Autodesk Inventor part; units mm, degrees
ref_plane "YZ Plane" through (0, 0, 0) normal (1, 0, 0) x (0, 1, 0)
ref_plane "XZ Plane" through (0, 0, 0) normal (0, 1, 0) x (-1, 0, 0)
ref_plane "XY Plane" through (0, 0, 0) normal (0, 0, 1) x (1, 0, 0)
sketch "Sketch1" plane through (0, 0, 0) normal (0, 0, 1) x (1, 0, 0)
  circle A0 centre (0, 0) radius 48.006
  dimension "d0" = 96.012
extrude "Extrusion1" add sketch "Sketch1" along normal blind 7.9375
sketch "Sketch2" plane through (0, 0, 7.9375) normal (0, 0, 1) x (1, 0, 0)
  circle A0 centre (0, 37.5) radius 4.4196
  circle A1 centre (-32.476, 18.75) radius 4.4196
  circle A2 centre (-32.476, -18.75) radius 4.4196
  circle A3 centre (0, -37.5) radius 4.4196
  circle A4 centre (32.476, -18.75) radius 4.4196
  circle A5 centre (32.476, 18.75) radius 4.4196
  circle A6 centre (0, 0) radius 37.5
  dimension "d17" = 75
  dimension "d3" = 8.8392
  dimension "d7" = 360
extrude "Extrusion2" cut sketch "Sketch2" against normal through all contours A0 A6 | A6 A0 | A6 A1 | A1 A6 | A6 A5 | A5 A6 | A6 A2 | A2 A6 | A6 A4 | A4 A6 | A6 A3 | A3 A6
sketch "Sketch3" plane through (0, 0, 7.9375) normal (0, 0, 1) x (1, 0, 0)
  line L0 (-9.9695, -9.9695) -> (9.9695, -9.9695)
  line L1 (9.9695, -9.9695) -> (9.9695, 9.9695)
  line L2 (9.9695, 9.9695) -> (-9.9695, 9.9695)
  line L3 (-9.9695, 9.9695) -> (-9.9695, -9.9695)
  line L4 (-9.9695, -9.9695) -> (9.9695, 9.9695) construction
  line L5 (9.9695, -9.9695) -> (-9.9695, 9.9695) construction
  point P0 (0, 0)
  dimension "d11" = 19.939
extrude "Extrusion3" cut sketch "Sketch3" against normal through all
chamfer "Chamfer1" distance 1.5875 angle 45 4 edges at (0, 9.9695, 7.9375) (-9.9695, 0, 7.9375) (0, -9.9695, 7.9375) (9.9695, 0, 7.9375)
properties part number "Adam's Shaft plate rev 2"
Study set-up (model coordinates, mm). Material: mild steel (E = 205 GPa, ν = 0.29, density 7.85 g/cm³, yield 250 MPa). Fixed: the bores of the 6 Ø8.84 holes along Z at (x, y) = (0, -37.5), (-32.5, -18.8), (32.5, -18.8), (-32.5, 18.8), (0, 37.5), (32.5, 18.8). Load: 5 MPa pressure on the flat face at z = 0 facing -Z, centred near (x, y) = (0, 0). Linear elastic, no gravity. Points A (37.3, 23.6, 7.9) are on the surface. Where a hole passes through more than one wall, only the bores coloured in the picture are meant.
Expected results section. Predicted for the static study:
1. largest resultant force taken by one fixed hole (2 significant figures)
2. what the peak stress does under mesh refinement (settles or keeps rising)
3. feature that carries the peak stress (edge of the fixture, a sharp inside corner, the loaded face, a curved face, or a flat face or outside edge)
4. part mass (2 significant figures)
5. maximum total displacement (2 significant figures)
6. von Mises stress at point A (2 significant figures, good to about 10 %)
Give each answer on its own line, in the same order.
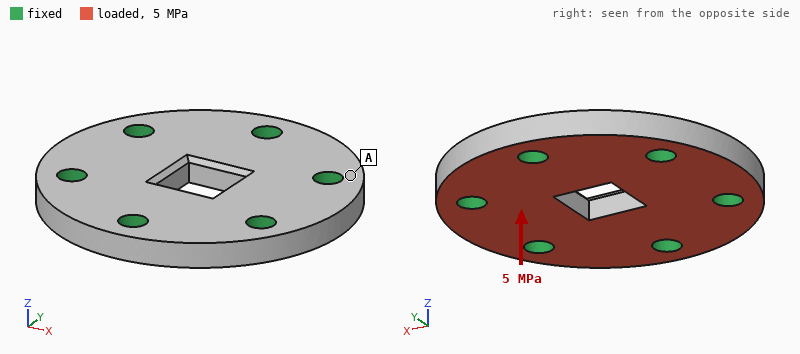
5.4 kN
keeps rising
edge of the fixture
400 g
16 µm
20 MPa
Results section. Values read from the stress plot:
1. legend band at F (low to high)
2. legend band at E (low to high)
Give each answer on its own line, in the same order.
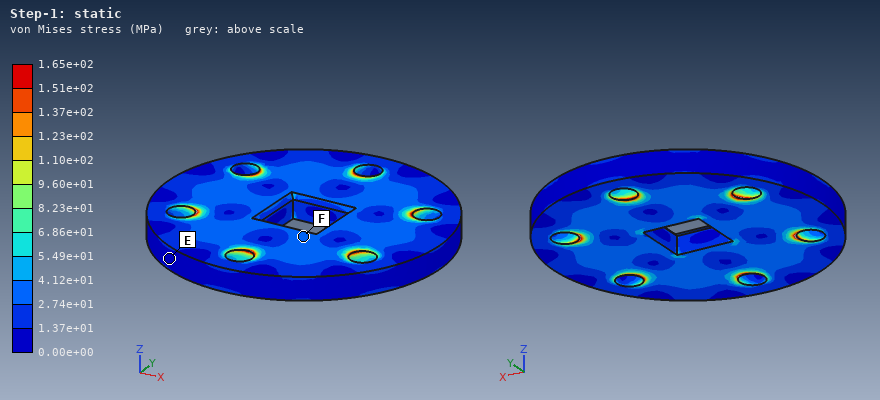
2.74e+01 to 4.12e+01 MPa
0.00e+00 to 1.37e+01 MPa
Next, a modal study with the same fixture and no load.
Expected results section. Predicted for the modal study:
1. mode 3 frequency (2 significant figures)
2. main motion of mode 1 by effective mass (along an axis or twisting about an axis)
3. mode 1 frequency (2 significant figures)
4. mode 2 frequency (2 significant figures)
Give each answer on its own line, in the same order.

21 kHz
along Z
14 kHz
21 kHz
